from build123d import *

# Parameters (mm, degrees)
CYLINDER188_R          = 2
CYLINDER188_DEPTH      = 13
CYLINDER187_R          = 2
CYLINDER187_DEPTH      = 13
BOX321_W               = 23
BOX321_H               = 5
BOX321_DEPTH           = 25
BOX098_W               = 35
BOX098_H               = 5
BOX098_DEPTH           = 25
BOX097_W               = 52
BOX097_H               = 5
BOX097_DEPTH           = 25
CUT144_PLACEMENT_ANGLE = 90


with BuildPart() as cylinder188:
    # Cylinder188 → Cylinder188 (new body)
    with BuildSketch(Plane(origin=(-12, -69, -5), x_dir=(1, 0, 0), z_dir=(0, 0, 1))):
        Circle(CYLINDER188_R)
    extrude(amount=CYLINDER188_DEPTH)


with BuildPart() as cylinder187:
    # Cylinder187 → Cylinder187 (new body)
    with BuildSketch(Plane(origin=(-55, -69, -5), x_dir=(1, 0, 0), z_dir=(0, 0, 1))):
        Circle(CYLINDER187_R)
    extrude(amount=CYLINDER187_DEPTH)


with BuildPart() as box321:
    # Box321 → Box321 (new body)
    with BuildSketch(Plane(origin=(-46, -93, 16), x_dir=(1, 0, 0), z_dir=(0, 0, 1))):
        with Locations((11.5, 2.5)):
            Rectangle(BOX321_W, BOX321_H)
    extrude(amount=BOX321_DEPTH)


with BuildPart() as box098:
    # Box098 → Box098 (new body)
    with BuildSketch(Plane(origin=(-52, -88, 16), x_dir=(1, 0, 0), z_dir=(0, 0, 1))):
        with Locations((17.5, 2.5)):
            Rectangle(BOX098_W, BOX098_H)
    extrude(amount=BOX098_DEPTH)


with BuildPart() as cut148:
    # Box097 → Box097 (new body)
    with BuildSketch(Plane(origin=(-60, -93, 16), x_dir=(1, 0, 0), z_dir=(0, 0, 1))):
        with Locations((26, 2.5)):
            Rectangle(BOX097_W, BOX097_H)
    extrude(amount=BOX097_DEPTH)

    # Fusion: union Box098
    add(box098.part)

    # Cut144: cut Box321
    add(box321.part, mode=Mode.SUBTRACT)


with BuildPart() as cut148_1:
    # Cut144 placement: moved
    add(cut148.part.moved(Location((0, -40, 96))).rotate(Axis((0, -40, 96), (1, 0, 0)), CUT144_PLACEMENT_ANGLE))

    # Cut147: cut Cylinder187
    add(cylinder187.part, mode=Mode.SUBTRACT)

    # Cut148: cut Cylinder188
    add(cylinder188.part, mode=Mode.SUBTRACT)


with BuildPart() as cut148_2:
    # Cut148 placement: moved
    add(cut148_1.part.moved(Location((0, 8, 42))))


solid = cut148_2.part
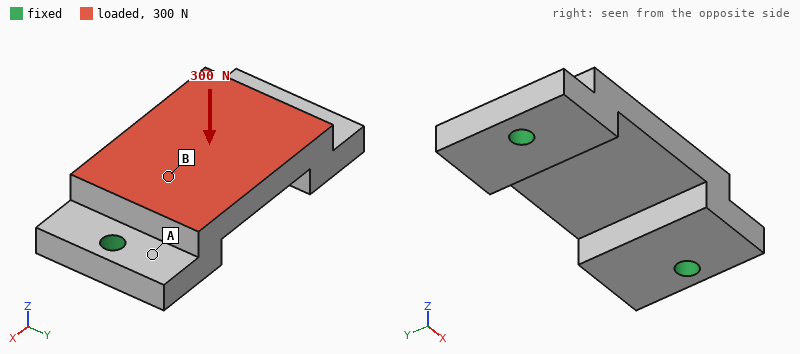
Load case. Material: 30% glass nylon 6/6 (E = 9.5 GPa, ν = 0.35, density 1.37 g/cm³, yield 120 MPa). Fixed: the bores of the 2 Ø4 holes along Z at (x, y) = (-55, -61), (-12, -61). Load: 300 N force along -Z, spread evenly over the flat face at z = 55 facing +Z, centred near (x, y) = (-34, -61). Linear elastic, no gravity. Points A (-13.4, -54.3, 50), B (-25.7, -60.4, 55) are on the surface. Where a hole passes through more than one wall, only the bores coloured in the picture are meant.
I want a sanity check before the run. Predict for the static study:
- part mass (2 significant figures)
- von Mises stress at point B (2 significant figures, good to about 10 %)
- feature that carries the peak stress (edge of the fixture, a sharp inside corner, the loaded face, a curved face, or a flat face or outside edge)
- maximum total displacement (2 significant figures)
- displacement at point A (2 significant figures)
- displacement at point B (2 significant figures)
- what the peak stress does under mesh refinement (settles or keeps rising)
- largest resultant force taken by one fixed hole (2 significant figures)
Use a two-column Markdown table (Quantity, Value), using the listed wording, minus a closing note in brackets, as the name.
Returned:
| Quantity | Value |
|---|---|
| part mass | 11 g |
| von Mises stress at point B | 3.0 MPa |
| feature that carries the peak stress | edge of the fixture |
| maximum total displacement | 26 µm |
| displacement at point A | 4.2 µm |
| displacement at point B | 16 µm |
| what the peak stress does under mesh refinement | keeps rising |
| largest resultant force taken by one fixed hole | 230 N |
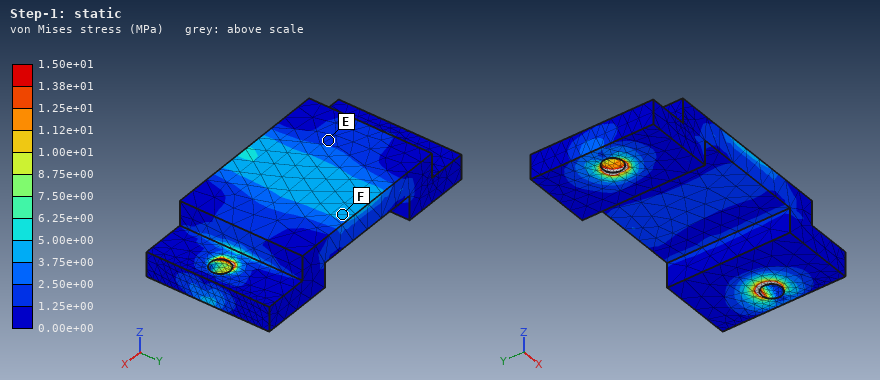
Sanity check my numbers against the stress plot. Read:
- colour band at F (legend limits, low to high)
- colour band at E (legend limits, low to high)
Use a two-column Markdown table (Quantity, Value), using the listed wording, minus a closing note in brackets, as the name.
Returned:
| Quantity | Value |
|---|---|
| colour band at F | 3.75e+00 to 5.00e+00 MPa |
| colour band at E | 1.25e+00 to 2.50e+00 MPa |
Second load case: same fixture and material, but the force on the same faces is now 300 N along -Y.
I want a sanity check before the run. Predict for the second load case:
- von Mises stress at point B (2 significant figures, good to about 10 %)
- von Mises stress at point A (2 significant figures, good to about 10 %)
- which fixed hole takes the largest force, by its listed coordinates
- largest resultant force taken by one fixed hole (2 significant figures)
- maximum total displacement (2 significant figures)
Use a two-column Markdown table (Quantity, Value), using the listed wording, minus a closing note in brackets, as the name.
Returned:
| Quantity | Value |
|---|---|
| von Mises stress at point B | 3.2 MPa |
| von Mises stress at point A | 5.9 MPa |
| which fixed hole takes the largest force, by its listed coordinates | (-55, -61) |
| largest resultant force taken by one fixed hole | 160 N |
| maximum total displacement | 53 µm |
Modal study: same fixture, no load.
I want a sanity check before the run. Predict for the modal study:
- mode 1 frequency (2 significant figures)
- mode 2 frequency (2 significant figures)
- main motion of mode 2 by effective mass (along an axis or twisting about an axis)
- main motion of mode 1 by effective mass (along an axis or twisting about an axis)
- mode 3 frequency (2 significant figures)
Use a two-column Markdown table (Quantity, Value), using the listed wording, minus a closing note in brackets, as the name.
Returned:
| Quantity | Value |
|---|---|
| mode 1 frequency | 5500 Hz |
| mode 2 frequency | 8100 Hz |
| main motion of mode 2 by effective mass | along Z |
| main motion of mode 1 by effective mass | along Y |
| mode 3 frequency | 10 kHz |
